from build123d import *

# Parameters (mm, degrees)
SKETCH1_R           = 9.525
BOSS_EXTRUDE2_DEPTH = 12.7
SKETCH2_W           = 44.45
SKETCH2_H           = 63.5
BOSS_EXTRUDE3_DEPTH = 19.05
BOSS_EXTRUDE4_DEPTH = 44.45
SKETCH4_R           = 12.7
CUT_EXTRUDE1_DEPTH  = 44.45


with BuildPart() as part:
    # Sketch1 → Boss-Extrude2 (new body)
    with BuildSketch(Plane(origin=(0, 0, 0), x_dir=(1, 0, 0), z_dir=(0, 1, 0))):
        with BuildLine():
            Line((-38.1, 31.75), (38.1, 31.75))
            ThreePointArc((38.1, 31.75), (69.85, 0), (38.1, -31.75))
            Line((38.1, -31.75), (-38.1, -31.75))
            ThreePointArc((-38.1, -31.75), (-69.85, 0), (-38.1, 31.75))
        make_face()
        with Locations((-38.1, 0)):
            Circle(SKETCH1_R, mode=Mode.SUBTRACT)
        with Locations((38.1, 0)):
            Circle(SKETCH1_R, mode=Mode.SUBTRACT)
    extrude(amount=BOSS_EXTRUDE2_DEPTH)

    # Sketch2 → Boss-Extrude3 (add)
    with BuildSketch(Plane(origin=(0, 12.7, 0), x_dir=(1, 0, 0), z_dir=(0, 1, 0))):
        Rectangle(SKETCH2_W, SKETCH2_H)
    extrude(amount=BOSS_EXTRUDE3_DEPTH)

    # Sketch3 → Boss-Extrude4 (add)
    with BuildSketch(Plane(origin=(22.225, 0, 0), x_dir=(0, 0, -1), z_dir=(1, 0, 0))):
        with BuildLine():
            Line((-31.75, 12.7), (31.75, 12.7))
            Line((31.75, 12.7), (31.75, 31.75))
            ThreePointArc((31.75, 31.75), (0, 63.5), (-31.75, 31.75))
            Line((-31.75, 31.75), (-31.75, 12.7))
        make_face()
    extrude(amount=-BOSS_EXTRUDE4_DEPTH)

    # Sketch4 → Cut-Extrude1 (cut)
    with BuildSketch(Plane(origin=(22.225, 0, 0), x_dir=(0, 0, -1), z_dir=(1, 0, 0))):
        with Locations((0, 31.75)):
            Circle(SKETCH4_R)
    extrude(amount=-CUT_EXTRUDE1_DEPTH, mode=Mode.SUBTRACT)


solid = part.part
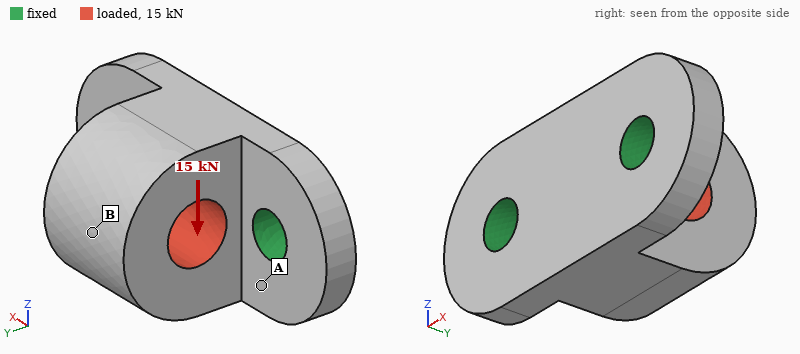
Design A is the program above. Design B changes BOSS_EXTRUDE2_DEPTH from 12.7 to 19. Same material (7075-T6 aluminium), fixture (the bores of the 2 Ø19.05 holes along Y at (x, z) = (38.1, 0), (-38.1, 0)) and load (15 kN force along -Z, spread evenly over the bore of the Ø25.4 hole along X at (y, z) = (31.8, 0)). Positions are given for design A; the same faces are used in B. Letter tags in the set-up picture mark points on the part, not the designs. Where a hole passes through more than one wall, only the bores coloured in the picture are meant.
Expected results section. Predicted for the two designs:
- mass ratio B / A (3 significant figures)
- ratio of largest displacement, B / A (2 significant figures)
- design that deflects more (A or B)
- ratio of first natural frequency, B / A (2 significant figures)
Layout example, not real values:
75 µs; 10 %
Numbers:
1.15; 0.44; A; 1.5
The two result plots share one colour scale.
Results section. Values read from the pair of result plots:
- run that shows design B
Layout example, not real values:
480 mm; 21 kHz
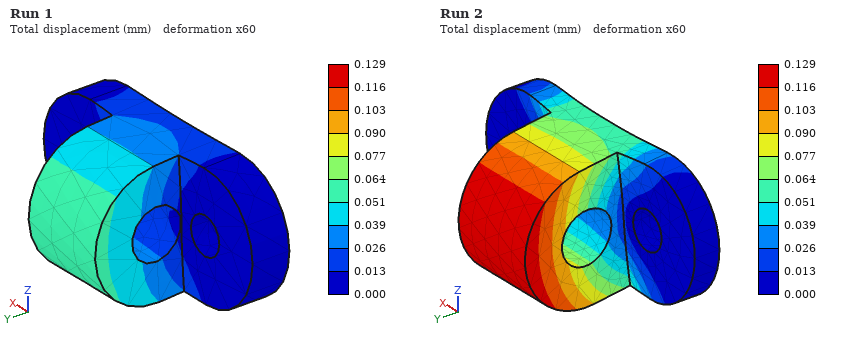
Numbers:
Run 1
